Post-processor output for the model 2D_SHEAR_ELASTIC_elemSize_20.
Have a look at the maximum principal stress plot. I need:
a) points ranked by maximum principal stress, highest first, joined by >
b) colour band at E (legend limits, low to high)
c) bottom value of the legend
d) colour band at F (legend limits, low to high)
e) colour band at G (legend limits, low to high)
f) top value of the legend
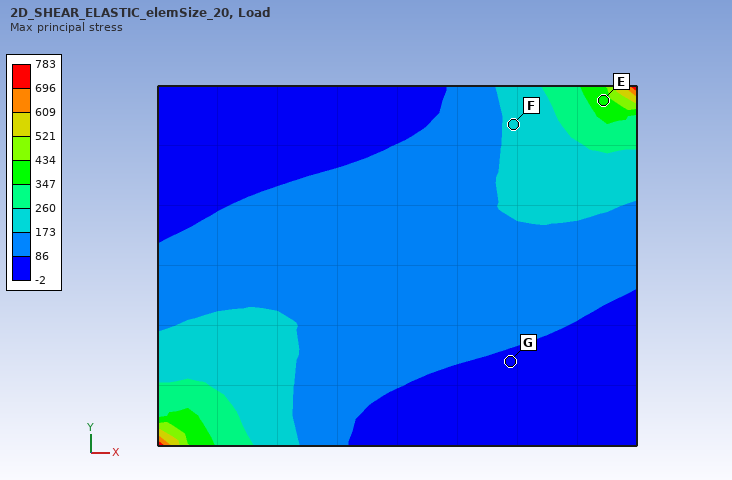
E > F > G
347 to 434
-2
173 to 260
-2 to 86
783
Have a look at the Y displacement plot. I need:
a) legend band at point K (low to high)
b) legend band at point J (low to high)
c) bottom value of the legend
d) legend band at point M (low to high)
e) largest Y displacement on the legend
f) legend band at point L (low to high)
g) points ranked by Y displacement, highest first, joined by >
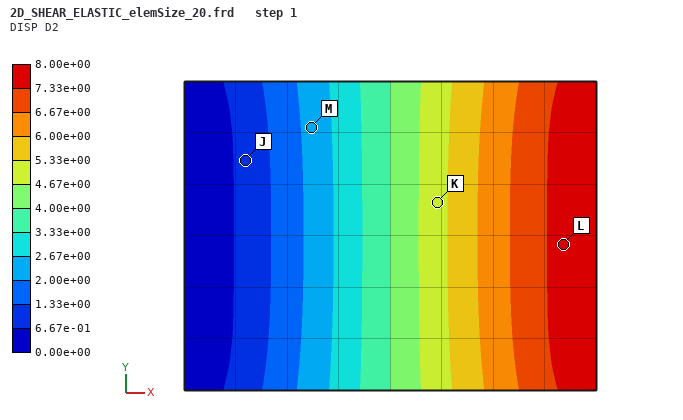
4.67e+00 to 5.33e+00
6.67e-01 to 1.33e+00
0.00e+00
2.00e+00 to 2.67e+00
8.00e+00
7.33e+00 to 8.00e+00
L > K > M > J
